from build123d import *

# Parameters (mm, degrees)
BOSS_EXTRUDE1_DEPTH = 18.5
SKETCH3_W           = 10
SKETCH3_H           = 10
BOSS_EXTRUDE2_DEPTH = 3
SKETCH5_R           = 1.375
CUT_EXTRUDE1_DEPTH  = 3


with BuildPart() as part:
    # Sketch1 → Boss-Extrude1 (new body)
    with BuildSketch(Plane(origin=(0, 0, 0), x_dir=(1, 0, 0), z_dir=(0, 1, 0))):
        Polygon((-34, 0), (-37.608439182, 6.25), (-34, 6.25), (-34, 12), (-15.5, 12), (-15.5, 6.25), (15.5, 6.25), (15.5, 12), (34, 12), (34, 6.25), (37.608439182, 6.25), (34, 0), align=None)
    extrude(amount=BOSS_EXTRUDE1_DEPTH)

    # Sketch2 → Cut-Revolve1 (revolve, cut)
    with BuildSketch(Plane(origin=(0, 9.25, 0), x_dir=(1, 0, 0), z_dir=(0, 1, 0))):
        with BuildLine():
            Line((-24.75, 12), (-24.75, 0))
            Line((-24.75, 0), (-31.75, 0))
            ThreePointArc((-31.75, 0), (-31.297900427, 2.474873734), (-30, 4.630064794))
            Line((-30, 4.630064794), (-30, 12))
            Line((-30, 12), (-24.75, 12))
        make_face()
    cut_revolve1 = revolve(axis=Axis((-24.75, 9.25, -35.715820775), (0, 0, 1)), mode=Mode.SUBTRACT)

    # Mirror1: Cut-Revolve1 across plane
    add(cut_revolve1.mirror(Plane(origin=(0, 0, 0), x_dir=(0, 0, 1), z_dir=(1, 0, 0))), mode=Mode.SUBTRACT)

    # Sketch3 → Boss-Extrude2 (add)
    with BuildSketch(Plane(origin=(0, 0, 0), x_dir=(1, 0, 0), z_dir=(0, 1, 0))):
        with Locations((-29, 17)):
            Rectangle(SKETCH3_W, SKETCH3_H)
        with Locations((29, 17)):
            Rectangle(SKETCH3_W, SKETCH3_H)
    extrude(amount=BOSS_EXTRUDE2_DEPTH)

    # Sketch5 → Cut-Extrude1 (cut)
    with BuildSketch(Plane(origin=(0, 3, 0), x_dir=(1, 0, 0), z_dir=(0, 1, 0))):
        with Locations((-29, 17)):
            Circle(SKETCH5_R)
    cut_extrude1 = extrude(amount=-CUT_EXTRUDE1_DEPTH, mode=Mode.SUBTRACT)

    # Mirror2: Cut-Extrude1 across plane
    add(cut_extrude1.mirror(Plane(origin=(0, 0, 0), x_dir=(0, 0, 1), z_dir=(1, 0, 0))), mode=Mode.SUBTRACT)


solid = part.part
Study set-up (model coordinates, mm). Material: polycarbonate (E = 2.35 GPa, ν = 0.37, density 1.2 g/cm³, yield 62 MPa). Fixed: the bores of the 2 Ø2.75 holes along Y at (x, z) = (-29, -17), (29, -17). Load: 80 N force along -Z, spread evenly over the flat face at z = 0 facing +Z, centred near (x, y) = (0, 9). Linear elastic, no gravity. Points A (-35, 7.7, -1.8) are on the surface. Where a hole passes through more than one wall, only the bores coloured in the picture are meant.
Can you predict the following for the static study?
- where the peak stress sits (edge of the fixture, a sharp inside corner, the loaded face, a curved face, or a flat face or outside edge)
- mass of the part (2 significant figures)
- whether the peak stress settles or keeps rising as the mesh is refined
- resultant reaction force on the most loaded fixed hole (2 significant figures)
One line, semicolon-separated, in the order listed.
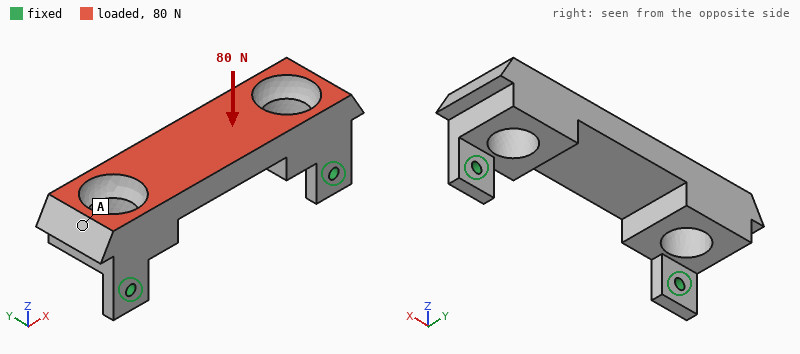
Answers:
edge of the fixture; 12 g; keeps rising; 49 N
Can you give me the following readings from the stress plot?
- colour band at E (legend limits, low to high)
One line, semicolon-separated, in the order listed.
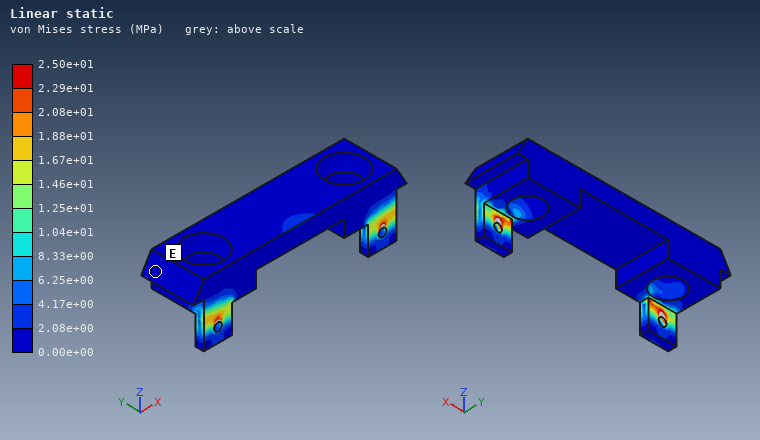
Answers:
0.00e+00 to 2.08e+00 MPa
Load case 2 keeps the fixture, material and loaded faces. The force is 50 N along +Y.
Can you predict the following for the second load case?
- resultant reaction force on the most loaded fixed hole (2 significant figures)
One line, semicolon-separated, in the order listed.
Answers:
25 N
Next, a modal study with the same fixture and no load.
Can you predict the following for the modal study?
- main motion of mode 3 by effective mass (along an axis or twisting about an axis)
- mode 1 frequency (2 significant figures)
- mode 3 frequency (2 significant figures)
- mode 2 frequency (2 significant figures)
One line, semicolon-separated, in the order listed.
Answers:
along X; 450 Hz; 2200 Hz; 1400 Hz
